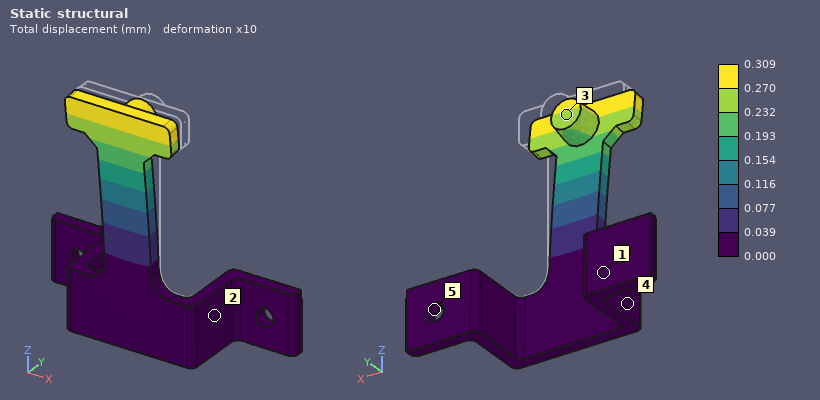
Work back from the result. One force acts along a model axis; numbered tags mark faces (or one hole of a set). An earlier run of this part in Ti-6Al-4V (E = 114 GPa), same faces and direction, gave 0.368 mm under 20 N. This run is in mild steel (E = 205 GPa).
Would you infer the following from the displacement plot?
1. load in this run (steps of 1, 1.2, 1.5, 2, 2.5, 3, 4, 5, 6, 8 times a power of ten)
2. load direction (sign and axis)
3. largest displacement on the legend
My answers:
30 N
-Y
0.309 mm
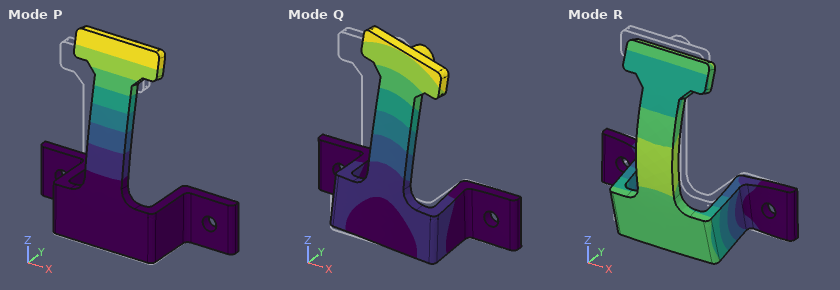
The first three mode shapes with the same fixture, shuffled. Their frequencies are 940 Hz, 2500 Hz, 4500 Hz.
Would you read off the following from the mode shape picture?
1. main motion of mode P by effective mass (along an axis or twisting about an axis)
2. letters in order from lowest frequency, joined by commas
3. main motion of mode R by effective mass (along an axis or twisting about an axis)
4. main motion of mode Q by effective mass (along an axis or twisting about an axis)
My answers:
along Y
P, Q, R
along Z
along X
